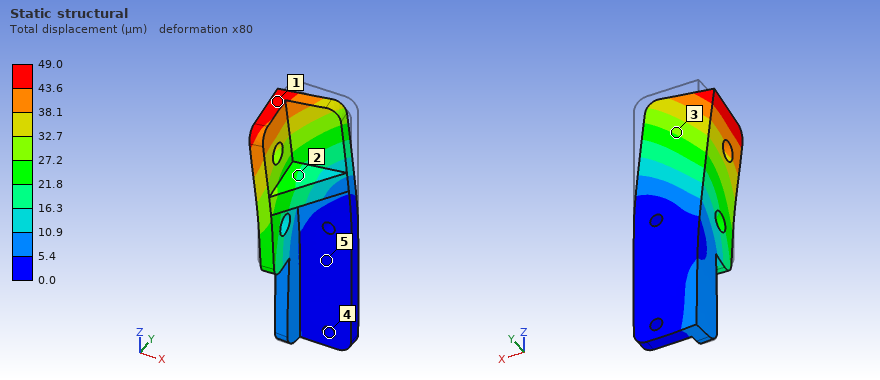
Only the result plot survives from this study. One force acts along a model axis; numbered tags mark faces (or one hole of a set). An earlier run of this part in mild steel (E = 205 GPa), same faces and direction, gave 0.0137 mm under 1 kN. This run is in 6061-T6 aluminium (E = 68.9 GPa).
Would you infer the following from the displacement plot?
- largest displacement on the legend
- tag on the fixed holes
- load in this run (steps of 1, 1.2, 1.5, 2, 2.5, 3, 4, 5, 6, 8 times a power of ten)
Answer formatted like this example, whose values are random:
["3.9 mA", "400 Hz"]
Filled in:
["49.0 µm", "4", "1.2 kN"]
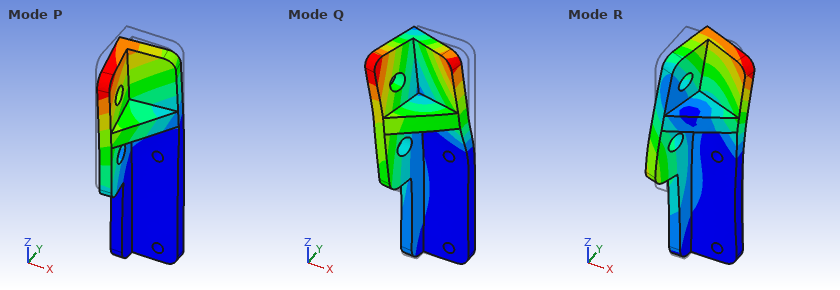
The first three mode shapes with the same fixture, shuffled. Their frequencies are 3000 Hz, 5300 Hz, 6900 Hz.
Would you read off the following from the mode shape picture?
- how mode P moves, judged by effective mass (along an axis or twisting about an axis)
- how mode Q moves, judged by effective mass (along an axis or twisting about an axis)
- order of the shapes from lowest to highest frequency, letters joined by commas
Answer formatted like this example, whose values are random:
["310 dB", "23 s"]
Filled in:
["along Y", "along X", "P, Q, R"]
